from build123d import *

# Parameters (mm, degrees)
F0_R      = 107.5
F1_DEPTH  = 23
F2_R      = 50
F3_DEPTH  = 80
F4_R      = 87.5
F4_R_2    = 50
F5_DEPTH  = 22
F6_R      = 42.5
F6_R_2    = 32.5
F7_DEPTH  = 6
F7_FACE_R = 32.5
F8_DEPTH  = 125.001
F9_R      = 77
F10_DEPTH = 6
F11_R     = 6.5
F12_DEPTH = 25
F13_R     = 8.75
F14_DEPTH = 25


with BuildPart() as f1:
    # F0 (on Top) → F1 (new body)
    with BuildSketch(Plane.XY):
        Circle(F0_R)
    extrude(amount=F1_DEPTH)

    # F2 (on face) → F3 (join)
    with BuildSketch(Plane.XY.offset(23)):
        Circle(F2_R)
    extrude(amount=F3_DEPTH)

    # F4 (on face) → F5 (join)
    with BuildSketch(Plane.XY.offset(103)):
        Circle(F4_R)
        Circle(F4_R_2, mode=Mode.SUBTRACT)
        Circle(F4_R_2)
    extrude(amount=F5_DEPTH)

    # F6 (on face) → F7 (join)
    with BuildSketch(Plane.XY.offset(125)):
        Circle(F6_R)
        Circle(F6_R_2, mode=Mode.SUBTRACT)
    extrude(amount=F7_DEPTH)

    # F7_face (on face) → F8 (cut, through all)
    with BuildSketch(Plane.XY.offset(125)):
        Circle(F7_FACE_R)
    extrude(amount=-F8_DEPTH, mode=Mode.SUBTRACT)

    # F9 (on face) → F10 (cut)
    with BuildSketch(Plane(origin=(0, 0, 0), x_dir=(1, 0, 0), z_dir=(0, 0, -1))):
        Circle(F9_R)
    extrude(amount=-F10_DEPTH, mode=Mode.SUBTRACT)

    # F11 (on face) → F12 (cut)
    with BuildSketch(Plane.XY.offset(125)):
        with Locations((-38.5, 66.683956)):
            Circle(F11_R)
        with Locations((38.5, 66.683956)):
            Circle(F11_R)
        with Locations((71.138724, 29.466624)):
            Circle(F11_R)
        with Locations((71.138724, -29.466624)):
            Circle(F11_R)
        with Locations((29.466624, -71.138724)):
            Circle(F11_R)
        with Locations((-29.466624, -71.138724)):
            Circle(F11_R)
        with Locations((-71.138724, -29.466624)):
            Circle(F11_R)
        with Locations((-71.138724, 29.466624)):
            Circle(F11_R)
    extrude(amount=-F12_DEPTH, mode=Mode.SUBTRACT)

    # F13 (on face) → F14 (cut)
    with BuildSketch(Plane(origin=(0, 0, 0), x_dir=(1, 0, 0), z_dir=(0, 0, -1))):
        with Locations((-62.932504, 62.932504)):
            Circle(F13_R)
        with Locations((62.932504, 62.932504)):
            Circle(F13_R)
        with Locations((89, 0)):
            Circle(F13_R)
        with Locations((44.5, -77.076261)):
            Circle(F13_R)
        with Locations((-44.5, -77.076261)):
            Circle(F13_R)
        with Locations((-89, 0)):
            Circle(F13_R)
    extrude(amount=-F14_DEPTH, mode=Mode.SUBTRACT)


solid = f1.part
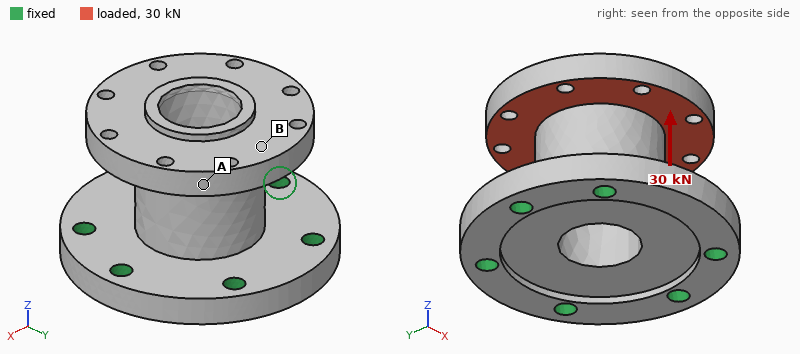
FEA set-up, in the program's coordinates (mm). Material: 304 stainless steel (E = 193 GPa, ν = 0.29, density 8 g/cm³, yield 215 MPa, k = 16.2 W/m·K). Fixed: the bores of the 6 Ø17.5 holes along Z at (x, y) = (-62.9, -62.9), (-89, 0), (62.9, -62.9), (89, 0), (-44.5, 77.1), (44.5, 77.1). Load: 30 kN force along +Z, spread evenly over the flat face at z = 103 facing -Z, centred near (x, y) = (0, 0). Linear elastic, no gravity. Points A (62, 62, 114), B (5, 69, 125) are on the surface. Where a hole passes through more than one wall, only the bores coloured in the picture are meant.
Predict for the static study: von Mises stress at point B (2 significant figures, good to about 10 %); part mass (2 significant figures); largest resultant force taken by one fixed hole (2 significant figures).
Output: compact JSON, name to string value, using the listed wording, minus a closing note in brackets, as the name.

{"von Mises stress at point B": "7.5 MPa", "part mass": "12 kg", "largest resultant force taken by one fixed hole": "6.3 kN"}
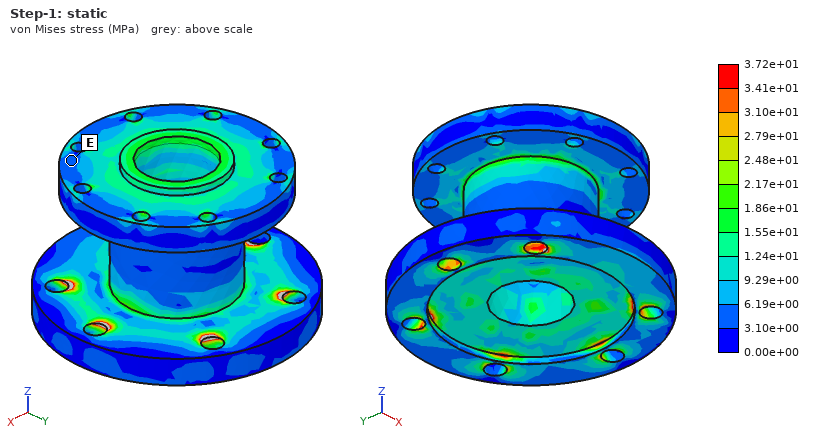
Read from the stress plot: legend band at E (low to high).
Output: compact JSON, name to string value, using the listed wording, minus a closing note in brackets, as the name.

{"legend band at E": "3.10e+00 to 6.19e+00 MPa"}
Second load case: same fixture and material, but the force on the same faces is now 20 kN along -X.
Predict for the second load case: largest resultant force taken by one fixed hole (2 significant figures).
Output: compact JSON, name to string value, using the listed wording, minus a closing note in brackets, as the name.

{"largest resultant force taken by one fixed hole": "9.1 kN"}
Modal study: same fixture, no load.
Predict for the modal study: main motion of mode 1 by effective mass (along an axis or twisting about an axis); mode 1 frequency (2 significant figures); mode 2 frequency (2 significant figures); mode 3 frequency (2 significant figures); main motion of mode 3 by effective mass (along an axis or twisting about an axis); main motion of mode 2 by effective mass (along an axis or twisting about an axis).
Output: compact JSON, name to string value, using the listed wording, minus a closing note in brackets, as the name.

{"main motion of mode 1 by effective mass": "along Y", "mode 1 frequency": "1400 Hz", "mode 2 frequency": "1500 Hz", "mode 3 frequency": "2800 Hz", "main motion of mode 3 by effective mass": "along Z", "main motion of mode 2 by effective mass": "along X"}
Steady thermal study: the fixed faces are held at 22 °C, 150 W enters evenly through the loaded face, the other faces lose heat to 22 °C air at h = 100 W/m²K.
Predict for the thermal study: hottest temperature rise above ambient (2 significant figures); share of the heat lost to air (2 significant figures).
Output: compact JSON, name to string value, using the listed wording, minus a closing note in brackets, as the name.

{"hottest temperature rise above ambient": "35 K", "share of the heat lost to air": "98 %"}
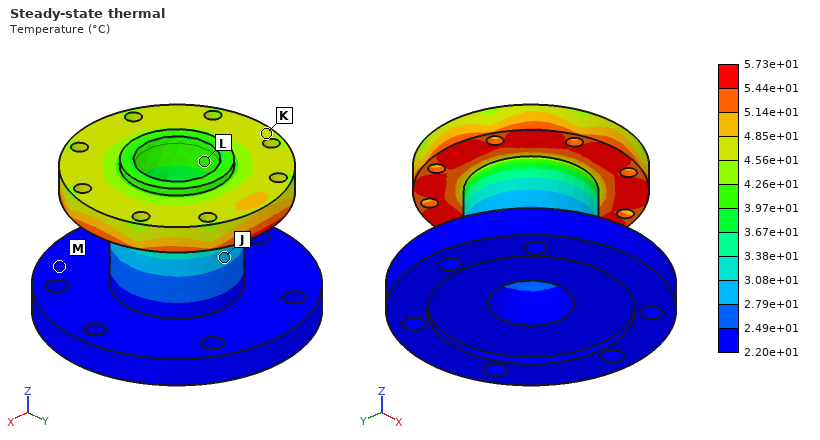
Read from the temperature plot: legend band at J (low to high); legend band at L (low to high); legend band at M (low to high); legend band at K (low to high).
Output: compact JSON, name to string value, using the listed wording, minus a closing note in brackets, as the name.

{"legend band at J": "2.79e+01 to 3.08e+01 °C", "legend band at L": "3.97e+01 to 4.26e+01 °C", "legend band at M": "2.20e+01 to 2.49e+01 °C", "legend band at K": "4.56e+01 to 4.85e+01 °C"}
